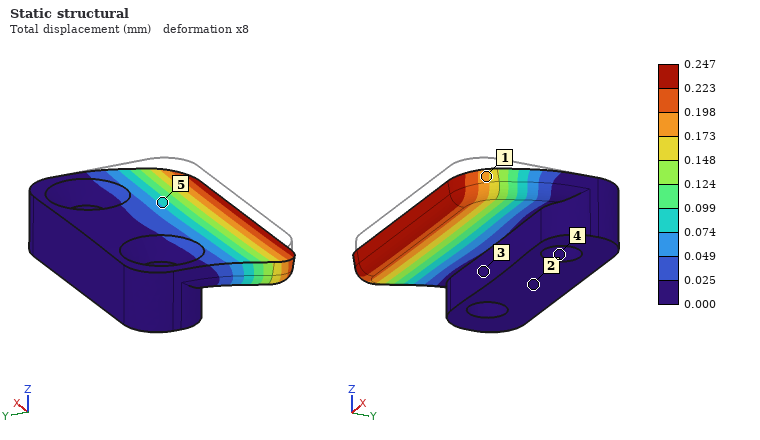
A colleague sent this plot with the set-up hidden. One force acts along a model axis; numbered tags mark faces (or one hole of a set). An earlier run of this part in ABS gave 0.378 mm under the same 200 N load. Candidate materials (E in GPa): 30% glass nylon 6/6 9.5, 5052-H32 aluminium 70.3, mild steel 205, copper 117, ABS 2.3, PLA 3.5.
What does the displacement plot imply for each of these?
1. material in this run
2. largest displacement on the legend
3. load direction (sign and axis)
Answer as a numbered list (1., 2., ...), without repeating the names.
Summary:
1. PLA
2. 0.247 mm
3. -Z
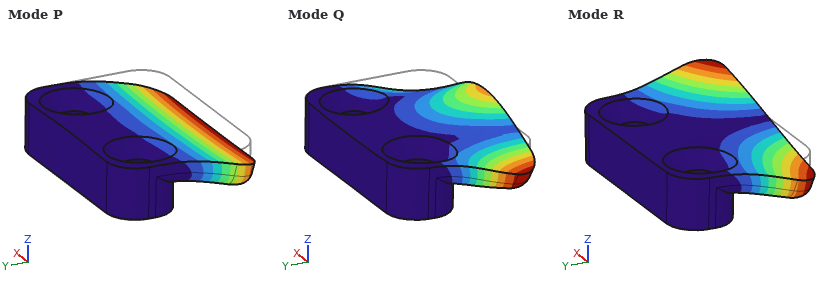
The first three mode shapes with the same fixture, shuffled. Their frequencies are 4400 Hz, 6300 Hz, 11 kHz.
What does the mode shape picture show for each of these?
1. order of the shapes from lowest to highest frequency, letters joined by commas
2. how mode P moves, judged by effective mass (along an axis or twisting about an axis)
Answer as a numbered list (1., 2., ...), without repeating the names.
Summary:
1. P, R, Q
2. along Z
